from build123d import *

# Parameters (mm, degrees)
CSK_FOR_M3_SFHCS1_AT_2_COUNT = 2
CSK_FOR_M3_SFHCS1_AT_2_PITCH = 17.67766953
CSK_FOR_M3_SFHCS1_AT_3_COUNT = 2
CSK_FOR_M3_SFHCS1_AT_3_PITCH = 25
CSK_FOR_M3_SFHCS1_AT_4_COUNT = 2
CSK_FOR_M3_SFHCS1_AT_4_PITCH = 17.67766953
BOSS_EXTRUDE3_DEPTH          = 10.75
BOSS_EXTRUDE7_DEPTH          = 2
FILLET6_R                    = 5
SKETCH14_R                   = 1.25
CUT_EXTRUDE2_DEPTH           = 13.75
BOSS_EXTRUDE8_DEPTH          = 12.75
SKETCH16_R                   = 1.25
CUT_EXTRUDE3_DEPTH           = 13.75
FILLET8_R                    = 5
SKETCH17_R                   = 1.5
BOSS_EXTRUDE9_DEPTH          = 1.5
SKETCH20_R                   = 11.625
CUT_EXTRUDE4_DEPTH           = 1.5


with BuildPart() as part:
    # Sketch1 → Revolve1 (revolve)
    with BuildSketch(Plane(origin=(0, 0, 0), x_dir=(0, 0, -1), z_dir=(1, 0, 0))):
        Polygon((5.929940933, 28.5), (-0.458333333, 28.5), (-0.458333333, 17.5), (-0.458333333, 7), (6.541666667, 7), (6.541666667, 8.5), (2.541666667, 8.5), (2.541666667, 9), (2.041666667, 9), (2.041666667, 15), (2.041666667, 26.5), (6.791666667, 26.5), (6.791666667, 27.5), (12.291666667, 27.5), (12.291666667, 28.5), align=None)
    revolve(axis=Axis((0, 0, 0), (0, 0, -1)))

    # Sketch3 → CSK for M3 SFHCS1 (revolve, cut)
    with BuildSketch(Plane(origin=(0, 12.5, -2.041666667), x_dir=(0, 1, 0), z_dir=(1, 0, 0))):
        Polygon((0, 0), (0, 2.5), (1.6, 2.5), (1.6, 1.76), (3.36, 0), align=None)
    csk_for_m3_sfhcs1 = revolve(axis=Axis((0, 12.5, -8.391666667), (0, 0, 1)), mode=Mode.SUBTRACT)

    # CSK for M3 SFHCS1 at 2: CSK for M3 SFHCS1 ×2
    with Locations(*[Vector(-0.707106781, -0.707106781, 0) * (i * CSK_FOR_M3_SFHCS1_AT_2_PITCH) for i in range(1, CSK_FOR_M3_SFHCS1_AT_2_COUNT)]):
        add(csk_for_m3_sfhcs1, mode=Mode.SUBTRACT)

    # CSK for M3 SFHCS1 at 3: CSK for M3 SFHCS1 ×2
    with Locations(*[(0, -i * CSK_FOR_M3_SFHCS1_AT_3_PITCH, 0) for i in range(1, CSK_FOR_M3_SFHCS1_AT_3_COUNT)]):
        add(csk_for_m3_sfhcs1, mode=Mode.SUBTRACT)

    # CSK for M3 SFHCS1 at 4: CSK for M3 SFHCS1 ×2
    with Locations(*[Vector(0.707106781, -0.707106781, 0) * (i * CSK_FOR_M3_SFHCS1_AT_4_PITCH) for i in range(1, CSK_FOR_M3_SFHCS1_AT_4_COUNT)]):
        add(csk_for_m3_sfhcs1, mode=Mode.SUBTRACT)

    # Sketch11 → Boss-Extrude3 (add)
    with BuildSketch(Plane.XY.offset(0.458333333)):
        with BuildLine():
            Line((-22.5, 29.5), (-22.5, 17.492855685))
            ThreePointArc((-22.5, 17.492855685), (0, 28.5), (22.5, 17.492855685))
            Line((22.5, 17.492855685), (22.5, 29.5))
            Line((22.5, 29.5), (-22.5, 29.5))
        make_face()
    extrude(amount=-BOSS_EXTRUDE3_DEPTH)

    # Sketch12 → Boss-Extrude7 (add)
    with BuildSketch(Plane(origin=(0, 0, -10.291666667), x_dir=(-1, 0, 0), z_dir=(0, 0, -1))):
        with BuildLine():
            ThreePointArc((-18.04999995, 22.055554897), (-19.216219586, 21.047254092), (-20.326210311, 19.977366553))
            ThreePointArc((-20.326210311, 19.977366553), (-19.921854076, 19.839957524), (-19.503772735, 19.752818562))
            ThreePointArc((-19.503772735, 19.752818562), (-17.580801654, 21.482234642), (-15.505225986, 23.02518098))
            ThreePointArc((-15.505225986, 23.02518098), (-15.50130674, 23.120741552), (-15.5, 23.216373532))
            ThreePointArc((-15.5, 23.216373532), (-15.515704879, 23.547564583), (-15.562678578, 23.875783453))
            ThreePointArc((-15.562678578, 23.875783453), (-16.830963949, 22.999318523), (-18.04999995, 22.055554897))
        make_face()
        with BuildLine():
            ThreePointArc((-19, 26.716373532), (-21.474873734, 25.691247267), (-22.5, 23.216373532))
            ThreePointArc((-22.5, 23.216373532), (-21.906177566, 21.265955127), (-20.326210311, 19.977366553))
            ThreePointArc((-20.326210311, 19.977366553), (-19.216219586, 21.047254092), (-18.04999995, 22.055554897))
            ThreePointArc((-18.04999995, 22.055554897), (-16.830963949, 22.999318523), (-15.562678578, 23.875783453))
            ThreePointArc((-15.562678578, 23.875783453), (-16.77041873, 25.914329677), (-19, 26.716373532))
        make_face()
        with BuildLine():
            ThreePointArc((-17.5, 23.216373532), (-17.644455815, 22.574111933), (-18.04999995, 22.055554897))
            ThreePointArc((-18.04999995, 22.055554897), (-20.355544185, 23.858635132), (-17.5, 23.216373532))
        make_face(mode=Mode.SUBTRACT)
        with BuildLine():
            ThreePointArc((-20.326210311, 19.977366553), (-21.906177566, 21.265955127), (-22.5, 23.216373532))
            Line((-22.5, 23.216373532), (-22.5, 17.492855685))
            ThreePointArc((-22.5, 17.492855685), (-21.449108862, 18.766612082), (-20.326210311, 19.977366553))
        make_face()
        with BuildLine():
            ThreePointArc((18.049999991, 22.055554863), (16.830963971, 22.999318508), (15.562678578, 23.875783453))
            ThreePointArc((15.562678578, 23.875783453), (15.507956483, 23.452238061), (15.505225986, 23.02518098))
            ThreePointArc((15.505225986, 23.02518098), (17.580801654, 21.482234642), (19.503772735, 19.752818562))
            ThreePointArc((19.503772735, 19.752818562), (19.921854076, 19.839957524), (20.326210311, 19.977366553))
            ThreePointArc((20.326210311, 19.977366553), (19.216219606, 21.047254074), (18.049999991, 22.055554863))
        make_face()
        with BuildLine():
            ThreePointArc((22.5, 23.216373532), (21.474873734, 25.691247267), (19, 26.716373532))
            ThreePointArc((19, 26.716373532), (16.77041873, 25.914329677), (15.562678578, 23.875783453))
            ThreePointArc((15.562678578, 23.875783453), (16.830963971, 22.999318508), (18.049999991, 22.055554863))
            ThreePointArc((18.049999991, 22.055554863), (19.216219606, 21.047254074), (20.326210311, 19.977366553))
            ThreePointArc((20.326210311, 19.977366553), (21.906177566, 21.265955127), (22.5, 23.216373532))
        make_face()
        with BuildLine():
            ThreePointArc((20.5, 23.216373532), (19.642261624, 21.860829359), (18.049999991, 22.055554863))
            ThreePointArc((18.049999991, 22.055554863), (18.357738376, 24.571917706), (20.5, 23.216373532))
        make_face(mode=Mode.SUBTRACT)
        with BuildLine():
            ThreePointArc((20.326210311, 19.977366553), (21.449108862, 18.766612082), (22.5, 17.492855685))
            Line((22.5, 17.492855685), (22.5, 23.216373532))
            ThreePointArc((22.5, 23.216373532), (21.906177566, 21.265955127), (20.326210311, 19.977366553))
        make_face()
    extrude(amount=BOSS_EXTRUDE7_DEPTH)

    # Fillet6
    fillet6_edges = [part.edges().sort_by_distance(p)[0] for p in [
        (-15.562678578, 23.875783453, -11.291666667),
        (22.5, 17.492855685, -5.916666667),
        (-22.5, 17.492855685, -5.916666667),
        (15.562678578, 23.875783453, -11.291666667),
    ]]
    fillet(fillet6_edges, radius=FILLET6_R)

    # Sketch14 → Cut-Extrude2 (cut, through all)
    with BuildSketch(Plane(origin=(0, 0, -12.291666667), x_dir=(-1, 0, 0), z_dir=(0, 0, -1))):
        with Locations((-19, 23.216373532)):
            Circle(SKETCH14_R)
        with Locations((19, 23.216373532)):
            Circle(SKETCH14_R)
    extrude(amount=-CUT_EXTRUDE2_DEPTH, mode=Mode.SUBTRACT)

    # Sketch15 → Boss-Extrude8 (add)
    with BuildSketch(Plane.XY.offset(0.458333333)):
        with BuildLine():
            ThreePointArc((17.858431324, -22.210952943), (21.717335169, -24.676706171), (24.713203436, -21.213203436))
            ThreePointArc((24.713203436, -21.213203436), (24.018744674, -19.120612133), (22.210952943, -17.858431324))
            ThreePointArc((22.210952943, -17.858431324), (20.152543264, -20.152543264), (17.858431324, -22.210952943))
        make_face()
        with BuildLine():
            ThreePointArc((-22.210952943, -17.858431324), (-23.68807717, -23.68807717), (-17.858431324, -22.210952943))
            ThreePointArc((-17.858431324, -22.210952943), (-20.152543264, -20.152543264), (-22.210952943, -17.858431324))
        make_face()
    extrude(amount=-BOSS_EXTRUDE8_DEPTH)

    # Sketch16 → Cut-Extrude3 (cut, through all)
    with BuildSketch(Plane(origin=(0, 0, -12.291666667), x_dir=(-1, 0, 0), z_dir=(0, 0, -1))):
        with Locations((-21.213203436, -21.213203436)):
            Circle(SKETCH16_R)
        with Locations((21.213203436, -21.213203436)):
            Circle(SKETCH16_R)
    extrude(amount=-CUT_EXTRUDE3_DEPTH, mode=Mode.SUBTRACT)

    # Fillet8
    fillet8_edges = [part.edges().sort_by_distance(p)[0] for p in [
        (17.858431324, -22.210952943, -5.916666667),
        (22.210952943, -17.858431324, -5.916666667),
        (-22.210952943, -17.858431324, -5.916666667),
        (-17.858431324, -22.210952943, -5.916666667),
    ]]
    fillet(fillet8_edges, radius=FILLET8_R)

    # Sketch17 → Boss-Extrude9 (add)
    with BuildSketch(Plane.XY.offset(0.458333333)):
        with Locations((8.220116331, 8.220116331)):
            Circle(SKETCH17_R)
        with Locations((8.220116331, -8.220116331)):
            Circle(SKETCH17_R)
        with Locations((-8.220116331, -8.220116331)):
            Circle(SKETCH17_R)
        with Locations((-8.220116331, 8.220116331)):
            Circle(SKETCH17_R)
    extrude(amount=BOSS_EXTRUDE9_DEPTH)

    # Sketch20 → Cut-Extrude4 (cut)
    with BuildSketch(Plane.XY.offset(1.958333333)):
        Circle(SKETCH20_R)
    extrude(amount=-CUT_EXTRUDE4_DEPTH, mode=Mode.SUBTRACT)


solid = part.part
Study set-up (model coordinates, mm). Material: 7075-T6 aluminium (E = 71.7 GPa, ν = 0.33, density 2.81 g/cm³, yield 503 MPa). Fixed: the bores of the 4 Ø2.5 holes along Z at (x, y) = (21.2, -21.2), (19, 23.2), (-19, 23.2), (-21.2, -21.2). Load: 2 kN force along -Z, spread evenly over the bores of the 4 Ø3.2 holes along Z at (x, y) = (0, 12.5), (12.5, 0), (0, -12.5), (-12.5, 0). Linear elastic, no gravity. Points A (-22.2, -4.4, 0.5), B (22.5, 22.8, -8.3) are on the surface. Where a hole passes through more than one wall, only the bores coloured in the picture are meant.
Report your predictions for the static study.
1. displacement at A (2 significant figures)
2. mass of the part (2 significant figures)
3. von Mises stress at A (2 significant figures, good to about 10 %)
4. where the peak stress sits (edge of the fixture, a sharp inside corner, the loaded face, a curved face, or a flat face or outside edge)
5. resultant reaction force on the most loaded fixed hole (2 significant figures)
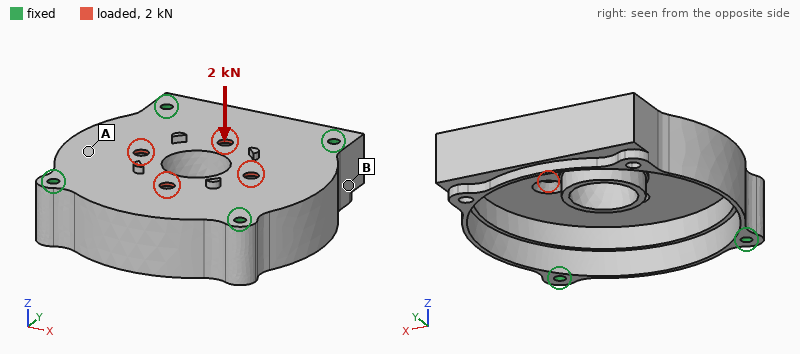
0.037 mm
33 g
68 MPa
the loaded face
520 N
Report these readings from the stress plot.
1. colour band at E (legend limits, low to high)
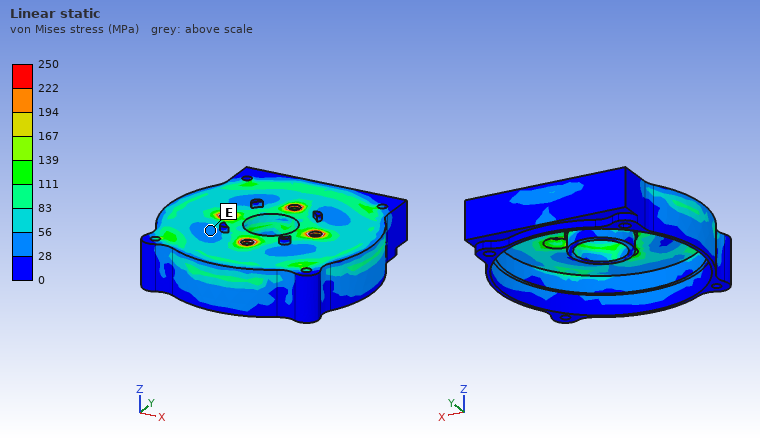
28 to 56 MPa
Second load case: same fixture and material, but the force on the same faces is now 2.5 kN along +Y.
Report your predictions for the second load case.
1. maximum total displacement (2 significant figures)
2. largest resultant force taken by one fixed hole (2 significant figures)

11 µm
680 N
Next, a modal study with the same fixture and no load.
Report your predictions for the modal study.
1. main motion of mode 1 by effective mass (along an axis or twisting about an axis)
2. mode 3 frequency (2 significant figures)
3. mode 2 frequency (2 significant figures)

along Z
13 kHz
13 kHz
